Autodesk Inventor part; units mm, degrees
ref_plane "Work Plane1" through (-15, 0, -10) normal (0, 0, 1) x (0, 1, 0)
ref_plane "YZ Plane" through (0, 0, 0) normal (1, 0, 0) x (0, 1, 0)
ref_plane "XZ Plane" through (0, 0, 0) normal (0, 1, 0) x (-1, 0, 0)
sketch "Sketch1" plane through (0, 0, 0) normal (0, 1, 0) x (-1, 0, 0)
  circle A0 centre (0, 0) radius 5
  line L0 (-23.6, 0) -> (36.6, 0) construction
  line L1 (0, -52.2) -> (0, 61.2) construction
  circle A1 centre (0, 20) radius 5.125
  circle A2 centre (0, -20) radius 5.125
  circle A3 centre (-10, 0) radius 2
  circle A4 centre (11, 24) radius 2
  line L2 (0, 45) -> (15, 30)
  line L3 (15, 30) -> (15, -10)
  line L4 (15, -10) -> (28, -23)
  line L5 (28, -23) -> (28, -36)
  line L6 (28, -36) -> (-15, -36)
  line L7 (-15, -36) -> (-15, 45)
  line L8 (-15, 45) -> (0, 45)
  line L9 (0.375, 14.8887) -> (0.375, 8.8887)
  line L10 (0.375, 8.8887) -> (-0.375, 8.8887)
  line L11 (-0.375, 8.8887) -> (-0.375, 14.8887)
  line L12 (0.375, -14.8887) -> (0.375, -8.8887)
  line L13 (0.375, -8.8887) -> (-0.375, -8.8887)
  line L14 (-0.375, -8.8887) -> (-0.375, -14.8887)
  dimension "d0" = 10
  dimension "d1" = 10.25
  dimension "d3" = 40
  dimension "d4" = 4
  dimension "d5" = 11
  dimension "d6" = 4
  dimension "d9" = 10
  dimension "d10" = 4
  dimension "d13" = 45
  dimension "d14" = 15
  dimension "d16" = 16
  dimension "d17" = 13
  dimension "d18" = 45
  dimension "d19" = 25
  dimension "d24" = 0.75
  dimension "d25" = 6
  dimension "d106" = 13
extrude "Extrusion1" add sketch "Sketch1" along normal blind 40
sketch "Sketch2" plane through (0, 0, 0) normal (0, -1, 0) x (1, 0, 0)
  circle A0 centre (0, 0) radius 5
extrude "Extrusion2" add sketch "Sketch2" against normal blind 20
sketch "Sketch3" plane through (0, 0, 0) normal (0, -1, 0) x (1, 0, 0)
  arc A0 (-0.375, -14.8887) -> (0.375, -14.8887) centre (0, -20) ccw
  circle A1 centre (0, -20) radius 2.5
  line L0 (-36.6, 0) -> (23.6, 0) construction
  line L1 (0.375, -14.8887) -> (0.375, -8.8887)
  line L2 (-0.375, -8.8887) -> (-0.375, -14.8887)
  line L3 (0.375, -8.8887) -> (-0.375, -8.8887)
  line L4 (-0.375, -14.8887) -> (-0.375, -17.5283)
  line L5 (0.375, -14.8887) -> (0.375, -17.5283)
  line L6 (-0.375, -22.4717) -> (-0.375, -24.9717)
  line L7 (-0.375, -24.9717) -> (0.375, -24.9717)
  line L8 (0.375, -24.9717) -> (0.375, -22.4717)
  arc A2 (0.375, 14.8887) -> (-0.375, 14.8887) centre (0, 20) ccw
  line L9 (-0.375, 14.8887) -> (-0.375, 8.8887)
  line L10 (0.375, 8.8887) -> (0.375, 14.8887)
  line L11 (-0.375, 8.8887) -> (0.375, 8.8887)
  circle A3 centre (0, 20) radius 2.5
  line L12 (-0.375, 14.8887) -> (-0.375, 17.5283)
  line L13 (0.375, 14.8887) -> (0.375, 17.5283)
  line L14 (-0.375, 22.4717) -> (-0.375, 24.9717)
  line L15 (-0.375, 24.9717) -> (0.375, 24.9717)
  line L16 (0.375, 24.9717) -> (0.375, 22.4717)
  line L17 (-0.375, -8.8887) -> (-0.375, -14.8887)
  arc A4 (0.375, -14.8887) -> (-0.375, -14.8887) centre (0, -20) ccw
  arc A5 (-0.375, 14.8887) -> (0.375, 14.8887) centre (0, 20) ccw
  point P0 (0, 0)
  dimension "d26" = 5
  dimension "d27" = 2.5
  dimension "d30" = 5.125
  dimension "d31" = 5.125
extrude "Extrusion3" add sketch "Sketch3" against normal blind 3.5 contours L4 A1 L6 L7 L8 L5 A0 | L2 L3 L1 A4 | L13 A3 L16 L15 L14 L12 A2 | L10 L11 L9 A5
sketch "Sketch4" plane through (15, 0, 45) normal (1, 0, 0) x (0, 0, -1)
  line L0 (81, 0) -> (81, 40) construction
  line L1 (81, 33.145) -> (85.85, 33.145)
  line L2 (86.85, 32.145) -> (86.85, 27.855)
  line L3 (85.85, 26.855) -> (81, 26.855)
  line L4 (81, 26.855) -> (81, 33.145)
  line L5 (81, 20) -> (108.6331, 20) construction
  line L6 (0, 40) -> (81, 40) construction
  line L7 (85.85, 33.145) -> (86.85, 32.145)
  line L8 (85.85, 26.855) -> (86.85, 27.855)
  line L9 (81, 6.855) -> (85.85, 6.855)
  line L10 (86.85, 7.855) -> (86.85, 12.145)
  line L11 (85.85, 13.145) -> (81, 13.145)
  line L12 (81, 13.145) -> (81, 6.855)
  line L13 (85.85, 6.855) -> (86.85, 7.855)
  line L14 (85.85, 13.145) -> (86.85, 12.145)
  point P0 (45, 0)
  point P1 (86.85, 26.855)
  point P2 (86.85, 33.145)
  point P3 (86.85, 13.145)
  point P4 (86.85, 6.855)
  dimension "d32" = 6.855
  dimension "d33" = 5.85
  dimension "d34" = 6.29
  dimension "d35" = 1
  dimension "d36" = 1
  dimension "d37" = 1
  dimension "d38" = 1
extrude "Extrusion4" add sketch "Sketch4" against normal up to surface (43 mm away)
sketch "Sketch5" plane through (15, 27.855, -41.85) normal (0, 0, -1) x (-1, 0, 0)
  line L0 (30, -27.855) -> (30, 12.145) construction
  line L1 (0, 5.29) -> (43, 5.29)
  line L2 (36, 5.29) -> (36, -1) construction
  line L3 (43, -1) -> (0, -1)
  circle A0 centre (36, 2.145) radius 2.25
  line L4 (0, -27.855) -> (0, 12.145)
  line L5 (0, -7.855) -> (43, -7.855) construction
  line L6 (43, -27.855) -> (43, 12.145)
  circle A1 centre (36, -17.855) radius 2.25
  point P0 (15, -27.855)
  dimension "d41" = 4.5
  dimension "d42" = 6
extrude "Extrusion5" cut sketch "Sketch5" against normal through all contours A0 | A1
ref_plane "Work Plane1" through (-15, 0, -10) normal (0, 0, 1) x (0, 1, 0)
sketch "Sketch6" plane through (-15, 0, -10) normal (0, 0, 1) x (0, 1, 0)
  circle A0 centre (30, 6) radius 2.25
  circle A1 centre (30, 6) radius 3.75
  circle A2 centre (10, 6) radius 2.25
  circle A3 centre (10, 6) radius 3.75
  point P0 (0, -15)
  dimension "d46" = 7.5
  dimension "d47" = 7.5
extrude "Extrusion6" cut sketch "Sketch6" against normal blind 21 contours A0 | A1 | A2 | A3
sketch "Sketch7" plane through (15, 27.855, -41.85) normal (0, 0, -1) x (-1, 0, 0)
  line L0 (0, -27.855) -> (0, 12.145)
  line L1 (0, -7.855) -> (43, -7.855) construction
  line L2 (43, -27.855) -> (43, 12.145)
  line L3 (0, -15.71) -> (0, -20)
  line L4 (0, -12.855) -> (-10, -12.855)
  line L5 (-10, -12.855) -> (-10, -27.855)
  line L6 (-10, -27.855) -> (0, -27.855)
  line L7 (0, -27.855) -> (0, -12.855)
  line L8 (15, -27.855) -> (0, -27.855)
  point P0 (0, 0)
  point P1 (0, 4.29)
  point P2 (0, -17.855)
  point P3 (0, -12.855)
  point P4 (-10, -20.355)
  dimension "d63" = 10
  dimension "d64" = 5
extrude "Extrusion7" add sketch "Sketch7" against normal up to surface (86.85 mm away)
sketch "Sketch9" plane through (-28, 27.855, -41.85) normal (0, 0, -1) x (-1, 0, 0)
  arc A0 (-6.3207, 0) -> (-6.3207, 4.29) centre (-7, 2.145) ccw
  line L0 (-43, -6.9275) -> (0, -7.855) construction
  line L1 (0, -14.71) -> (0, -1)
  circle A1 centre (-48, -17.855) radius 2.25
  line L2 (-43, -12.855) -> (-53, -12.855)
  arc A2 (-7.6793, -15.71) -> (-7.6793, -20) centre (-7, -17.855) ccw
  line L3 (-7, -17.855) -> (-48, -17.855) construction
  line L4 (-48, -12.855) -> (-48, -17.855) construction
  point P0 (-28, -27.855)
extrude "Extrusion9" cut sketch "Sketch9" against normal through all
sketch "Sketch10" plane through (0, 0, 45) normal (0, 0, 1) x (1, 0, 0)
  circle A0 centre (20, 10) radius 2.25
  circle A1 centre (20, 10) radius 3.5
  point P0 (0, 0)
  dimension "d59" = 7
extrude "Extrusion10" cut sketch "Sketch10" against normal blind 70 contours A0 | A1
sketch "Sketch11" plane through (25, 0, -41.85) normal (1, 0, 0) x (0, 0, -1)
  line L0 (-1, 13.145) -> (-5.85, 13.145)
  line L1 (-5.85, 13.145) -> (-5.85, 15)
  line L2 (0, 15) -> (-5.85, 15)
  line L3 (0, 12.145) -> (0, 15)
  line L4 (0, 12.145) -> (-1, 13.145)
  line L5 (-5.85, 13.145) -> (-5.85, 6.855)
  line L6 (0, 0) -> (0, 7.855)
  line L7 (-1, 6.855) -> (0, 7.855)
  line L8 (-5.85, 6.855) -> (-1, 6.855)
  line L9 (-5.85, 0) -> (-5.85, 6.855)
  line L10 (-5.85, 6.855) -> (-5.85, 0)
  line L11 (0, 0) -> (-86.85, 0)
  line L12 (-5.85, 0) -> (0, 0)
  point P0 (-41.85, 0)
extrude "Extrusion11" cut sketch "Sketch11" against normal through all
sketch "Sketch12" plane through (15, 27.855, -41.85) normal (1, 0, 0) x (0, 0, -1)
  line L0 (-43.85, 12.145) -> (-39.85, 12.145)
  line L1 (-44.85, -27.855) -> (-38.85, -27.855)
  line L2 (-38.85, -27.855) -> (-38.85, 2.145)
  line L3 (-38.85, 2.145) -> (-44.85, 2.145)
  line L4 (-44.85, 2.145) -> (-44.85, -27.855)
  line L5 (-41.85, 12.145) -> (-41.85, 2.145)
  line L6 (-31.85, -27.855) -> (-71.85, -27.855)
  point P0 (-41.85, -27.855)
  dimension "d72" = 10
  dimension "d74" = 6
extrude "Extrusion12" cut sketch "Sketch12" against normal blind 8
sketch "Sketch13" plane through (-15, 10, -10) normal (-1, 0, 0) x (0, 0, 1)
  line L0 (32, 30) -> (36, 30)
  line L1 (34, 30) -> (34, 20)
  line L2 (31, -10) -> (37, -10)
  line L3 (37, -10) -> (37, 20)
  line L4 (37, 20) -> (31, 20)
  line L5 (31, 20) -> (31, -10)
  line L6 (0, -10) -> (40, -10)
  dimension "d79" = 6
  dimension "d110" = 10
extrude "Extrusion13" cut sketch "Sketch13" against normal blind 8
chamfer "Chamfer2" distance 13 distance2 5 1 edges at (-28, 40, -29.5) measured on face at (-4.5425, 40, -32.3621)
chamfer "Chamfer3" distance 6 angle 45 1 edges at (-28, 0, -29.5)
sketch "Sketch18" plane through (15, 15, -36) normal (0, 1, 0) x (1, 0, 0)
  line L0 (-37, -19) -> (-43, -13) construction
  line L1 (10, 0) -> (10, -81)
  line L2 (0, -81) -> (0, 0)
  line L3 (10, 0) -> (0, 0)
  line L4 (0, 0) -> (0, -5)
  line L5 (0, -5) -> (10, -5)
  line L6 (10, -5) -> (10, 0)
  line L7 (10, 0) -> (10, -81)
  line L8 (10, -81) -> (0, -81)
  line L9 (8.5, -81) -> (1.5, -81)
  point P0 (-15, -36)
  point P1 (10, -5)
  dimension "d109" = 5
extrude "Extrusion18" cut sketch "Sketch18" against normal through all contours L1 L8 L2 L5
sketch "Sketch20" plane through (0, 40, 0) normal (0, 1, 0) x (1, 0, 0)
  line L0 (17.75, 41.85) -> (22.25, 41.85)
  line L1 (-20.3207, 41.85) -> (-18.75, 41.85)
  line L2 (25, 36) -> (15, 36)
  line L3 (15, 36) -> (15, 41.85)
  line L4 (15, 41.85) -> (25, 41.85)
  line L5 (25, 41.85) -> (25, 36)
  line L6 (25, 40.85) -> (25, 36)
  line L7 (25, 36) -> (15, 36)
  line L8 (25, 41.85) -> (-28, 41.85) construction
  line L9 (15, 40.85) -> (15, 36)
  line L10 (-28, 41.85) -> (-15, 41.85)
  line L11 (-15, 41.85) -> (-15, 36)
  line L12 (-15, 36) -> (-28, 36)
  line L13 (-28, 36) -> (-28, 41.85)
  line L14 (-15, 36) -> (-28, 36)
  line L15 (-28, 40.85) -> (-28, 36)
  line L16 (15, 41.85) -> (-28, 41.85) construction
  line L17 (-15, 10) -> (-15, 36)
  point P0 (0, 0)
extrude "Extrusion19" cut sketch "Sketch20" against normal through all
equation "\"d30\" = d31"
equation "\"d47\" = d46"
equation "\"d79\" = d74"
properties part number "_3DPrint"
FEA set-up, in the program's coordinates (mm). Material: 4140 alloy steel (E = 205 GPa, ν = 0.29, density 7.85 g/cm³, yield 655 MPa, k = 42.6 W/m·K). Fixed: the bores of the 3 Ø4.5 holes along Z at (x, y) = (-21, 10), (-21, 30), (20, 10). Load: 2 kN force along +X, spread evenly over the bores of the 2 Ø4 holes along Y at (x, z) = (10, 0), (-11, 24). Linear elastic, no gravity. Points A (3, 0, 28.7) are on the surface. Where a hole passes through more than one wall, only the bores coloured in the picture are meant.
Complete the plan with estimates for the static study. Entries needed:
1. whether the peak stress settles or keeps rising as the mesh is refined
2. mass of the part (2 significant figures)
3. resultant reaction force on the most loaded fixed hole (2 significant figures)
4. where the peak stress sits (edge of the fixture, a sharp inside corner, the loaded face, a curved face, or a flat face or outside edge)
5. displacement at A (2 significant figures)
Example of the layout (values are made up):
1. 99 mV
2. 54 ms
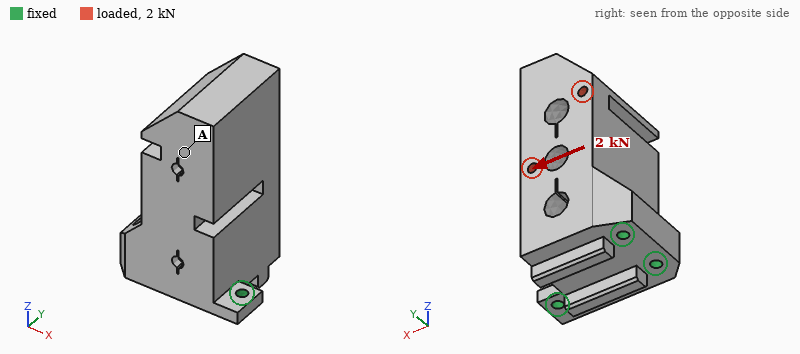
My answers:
1. keeps rising
2. 720 g
3. 2.4 kN
4. edge of the fixture
5. 15 µm
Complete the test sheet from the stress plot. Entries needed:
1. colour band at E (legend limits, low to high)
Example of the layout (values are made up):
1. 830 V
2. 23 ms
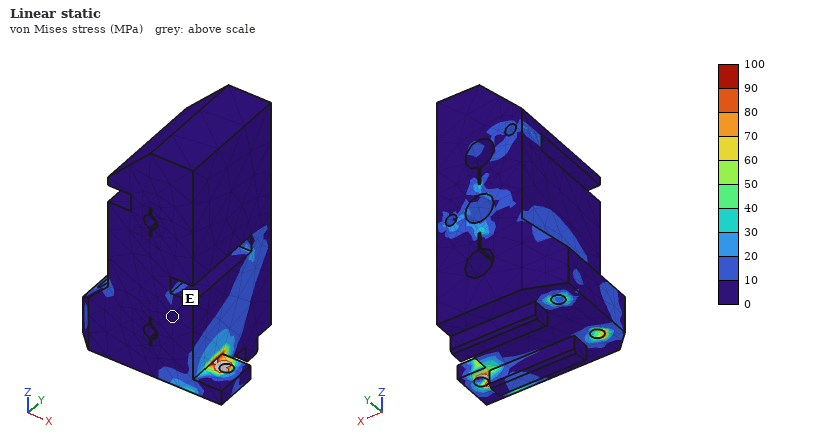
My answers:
1. 0 to 10 MPa
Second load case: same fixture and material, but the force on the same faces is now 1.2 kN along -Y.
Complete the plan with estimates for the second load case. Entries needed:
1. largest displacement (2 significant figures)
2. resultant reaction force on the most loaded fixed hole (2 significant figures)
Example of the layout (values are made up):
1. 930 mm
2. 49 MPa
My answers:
1. 20 µm
2. 2.5 kN
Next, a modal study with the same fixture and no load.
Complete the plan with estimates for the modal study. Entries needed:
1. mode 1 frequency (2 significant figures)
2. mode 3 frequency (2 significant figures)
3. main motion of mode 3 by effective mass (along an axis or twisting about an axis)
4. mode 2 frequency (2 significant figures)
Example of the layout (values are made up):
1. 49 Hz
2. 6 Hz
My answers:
1. 2000 Hz
2. 7800 Hz
3. twisting about Z
4. 2800 Hz
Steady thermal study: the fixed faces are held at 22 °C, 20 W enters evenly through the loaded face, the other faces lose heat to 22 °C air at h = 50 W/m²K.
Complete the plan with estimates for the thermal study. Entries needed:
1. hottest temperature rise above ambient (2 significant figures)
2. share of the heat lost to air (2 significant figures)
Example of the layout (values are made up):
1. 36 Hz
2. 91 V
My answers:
1. 29 K
2. 55 %
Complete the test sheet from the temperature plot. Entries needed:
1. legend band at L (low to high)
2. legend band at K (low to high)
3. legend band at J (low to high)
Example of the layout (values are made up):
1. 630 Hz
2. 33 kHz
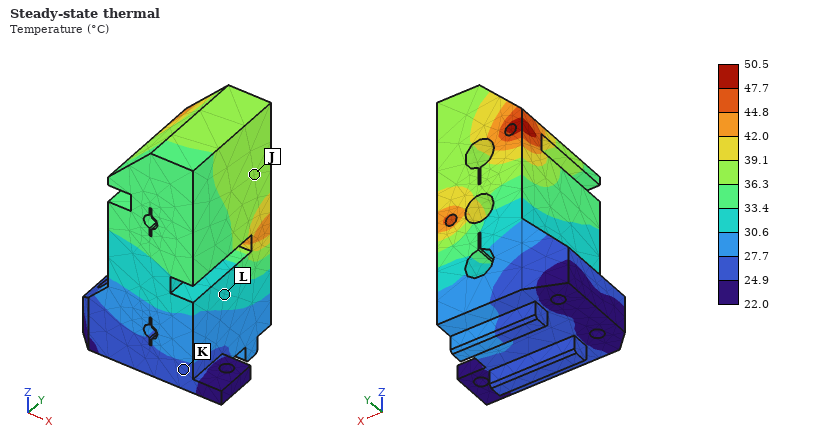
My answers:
1. 30.6 to 33.4 °C
2. 24.9 to 27.7 °C
3. 36.3 to 39.1 °C
